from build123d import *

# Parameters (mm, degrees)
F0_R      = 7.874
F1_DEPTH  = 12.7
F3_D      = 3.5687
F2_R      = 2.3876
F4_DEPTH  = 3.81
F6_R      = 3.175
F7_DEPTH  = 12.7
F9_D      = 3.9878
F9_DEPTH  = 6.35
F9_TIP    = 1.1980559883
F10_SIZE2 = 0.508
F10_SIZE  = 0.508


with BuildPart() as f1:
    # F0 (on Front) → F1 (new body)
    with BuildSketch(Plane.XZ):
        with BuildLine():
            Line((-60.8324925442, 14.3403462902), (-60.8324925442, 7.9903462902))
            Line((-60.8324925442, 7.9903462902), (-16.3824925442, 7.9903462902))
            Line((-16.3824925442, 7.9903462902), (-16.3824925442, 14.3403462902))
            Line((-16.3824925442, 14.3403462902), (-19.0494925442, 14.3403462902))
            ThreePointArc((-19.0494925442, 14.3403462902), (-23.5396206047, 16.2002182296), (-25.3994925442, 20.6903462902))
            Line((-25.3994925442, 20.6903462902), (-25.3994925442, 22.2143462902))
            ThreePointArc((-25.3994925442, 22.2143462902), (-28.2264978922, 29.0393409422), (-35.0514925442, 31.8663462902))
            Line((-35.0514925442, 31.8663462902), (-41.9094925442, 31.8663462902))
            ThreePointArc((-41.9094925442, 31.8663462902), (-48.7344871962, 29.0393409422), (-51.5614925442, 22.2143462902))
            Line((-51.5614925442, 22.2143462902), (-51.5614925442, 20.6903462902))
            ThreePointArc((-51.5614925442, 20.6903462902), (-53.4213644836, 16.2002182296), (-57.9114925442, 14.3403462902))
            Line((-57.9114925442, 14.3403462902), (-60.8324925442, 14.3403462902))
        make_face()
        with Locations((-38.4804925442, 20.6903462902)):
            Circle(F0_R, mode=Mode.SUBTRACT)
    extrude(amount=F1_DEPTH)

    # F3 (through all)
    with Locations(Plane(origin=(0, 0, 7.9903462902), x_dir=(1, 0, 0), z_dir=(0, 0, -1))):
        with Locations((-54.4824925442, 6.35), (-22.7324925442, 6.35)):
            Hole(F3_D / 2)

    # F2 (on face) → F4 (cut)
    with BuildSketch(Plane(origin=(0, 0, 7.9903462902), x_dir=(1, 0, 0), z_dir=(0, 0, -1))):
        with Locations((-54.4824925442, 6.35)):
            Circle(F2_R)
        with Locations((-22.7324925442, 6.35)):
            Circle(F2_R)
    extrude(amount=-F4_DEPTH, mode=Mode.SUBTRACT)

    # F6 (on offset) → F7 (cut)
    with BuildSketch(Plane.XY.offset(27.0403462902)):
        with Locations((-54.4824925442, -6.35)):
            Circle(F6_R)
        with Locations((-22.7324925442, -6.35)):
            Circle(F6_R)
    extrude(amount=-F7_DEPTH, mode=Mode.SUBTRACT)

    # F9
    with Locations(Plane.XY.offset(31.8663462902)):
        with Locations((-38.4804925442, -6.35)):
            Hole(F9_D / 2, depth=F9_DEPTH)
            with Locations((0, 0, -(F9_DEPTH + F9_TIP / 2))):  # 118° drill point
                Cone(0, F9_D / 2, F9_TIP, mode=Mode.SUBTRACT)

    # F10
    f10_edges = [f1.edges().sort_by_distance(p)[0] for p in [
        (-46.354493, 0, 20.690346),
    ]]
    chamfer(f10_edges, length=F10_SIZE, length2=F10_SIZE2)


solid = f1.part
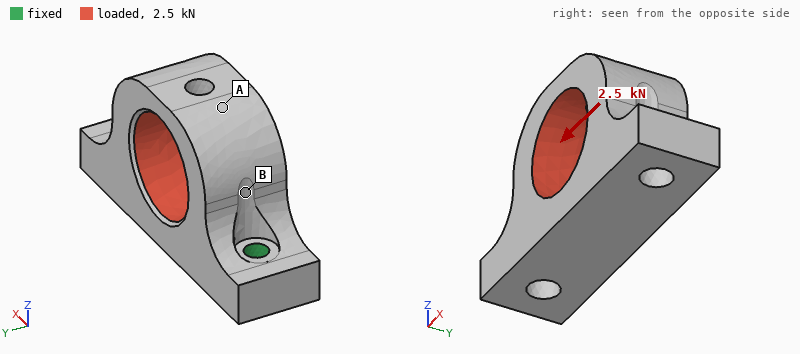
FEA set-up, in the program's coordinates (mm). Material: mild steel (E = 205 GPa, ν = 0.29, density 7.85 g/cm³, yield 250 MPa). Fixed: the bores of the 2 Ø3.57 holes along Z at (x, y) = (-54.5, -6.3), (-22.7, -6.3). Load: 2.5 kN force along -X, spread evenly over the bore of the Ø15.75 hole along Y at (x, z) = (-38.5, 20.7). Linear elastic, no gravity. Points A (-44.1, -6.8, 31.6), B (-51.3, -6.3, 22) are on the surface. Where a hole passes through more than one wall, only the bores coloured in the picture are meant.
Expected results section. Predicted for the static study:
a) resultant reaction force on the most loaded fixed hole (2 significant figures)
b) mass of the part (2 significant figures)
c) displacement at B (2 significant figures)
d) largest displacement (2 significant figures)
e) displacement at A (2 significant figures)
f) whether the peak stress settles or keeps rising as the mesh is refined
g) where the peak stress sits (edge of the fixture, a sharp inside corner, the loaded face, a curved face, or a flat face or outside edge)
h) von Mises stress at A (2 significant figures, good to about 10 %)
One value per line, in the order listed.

1.4 kN
50 g
4.2 µm
7.2 µm
6.8 µm
keeps rising
edge of the fixture
19 MPa
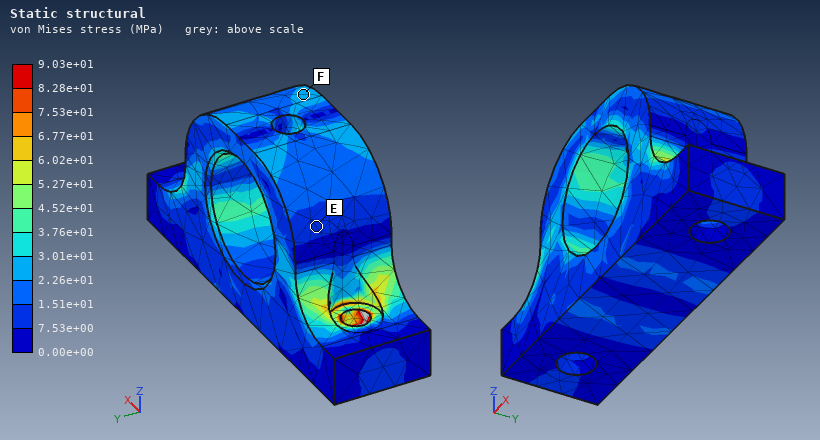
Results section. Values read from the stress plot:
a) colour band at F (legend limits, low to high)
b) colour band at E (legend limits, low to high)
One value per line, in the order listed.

2.26e+01 to 3.01e+01 MPa
7.53e+00 to 1.51e+01 MPa
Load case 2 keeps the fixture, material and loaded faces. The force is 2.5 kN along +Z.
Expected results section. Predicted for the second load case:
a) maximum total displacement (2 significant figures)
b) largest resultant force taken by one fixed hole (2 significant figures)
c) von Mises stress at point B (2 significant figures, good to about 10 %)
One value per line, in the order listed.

5.6 µm
1.3 kN
20 MPa
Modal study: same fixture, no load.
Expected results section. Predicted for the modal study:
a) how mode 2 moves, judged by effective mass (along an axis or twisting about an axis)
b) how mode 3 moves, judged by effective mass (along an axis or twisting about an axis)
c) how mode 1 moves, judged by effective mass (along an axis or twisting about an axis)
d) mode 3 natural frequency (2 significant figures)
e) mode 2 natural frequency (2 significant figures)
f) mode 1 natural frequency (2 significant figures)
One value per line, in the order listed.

along X
along Z
along Y
21 kHz
19 kHz
7700 Hz
